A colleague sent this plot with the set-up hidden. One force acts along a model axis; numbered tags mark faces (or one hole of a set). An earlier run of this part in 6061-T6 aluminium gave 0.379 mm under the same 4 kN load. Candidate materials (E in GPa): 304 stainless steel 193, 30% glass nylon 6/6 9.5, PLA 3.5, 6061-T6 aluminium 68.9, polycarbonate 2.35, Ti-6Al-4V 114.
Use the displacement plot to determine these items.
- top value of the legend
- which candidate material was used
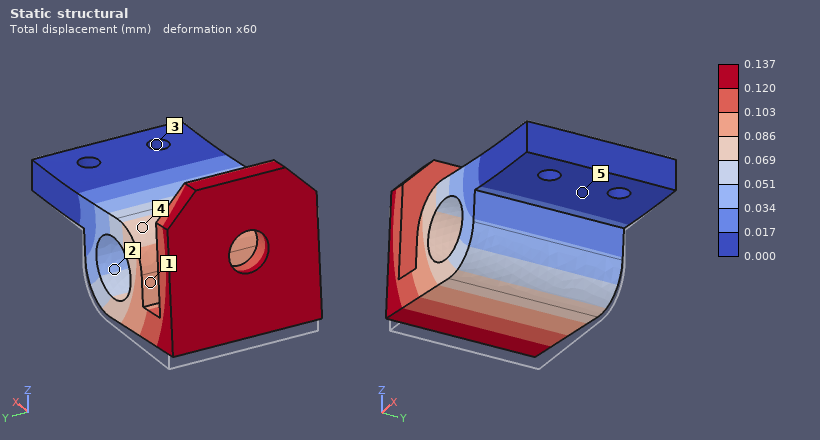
0.137 mm
304 stainless steel
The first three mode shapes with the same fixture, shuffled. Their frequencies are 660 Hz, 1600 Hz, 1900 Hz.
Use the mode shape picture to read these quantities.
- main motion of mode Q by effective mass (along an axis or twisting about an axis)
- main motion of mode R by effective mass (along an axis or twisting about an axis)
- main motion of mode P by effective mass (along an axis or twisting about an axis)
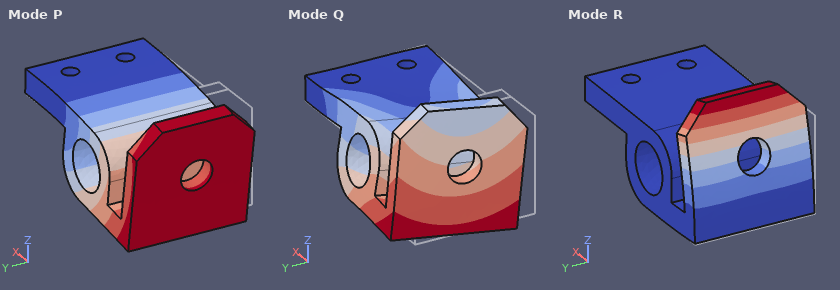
along Y
along X
along Z
